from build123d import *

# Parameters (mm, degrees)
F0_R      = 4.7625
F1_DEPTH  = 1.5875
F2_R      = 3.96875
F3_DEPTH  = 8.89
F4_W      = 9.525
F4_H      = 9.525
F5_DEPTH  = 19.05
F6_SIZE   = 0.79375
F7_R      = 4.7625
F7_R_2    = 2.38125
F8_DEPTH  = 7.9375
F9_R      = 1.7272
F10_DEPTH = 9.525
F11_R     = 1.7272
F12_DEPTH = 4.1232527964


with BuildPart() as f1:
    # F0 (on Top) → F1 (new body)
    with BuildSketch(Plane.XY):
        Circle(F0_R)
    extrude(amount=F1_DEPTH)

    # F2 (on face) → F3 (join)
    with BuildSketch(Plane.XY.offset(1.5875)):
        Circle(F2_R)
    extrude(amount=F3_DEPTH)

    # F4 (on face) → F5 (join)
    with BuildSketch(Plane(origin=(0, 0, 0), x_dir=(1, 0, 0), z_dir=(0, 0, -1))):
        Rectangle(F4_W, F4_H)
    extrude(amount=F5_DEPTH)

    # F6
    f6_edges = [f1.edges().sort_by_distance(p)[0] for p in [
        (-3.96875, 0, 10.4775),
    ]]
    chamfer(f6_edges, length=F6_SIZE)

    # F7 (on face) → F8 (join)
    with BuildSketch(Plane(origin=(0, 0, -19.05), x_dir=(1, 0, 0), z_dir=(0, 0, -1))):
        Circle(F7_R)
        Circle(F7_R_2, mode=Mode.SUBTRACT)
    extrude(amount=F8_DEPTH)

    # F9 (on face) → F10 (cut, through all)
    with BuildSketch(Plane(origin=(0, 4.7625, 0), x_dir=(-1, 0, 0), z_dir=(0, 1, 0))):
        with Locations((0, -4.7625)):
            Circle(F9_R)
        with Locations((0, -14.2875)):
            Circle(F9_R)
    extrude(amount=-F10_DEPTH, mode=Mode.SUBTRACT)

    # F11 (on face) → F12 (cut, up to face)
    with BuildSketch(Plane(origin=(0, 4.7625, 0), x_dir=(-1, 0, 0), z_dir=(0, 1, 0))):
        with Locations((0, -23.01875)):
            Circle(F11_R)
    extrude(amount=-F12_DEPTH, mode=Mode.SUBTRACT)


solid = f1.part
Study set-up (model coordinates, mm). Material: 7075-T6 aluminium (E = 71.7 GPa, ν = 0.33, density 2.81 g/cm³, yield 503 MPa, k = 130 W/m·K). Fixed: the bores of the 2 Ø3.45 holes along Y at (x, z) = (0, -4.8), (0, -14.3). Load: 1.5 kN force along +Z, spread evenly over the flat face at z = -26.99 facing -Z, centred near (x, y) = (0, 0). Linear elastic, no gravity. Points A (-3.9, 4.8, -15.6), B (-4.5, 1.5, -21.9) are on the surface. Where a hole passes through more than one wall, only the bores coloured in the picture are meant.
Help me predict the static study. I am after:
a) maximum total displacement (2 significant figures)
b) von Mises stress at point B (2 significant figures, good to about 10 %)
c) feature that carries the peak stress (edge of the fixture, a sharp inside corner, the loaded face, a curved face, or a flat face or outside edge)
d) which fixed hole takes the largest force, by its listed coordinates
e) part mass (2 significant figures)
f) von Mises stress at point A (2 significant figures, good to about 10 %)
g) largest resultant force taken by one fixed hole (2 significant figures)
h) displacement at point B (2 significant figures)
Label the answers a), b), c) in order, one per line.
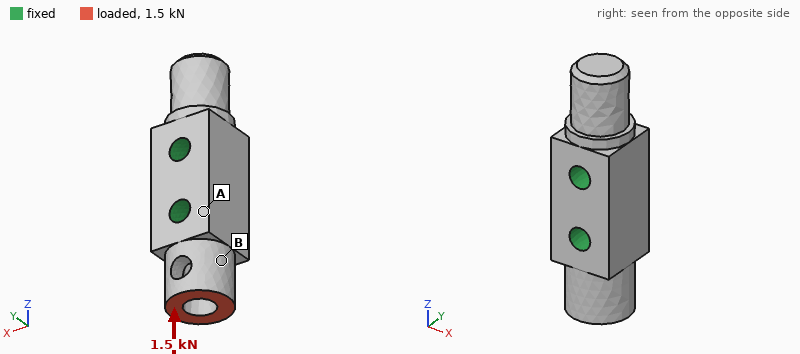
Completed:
a) 8.7 µm
b) 27 MPa
c) a curved face
d) (0, -14.3)
e) 7.0 g
f) 8.5 MPa
g) 1.3 kN
h) 3.2 µm
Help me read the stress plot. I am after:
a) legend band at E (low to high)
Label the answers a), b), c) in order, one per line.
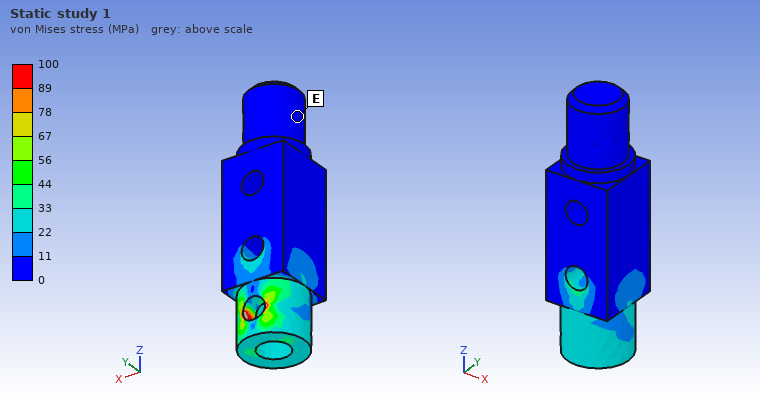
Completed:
a) 0 to 11 MPa
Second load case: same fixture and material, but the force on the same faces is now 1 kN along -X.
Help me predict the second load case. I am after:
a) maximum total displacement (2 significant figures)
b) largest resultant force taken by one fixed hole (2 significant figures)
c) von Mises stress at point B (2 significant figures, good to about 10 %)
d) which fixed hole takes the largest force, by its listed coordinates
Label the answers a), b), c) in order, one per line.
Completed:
a) 45 µm
b) 1.5 kN
c) 91 MPa
d) (0, -14.3)
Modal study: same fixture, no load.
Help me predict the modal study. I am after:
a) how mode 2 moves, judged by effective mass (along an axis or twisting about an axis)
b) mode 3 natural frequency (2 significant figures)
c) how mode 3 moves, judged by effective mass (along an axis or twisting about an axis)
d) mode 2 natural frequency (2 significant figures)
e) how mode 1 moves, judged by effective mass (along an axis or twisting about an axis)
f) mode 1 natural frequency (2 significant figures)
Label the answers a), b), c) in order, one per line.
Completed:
a) along Y
b) 36 kHz
c) along X
d) 33 kHz
e) along X
f) 28 kHz
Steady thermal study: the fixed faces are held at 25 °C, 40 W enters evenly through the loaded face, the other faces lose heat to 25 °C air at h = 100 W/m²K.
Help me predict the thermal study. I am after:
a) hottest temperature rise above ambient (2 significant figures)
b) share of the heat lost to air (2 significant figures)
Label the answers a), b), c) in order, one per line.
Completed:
a) 70 K
b) 4.1 %
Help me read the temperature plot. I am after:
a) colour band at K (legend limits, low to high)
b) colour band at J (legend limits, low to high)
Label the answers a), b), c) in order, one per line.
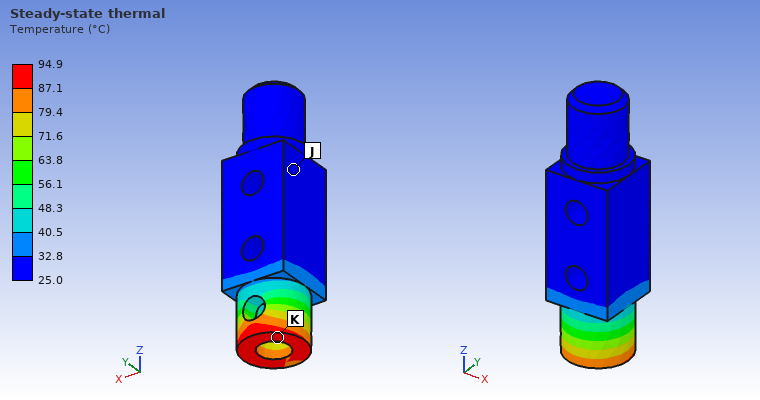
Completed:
a) 87.1 to 94.9 °C
b) 25.0 to 32.8 °C
